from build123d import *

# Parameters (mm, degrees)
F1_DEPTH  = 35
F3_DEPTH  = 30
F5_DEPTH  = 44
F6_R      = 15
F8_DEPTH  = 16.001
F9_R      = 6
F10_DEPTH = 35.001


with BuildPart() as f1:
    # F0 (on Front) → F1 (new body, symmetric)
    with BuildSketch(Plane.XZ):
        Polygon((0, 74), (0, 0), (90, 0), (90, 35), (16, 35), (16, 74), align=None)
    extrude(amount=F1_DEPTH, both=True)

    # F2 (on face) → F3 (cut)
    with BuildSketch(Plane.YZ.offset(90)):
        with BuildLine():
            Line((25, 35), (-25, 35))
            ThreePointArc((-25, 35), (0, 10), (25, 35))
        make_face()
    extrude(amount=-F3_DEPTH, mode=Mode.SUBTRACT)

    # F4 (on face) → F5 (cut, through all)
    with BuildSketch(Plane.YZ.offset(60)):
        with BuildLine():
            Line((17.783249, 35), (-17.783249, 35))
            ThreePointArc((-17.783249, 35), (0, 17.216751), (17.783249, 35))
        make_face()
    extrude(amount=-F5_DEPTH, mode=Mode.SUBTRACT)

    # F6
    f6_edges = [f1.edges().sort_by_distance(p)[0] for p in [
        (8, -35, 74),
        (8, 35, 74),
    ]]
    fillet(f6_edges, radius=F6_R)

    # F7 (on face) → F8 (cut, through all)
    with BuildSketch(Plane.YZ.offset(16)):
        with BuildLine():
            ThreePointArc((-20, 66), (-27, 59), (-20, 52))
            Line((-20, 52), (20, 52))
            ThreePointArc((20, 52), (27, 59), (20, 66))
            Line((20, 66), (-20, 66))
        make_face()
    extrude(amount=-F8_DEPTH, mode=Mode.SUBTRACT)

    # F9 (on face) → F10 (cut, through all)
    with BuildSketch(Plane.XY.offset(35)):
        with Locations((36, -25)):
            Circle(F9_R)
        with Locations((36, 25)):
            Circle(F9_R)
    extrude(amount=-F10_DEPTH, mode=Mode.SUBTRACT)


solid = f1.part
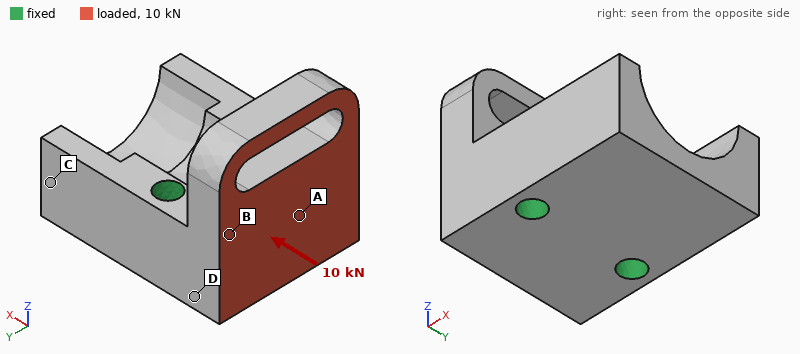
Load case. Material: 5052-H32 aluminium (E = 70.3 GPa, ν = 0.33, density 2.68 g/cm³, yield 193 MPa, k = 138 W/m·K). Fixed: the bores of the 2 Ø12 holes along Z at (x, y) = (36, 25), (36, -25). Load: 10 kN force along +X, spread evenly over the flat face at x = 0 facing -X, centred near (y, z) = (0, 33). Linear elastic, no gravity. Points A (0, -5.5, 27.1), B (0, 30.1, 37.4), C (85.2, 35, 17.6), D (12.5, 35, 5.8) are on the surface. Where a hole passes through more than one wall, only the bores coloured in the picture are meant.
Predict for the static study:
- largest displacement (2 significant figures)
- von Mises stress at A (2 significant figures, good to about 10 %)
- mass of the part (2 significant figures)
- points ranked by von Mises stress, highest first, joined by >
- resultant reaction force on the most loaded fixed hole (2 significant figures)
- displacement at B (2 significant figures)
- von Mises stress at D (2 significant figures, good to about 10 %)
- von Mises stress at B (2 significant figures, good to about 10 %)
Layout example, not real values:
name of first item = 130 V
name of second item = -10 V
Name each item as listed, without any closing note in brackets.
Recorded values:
largest displacement = 0.10 mm
von Mises stress at A = 16 MPa
mass of the part = 510 g
points ranked by von Mises stress, highest first, joined by > = B > A > D > C
resultant reaction force on the most loaded fixed hole = 5.1 kN
displacement at B = 0.019 mm
von Mises stress at D = 7.6 MPa
von Mises stress at B = 31 MPa
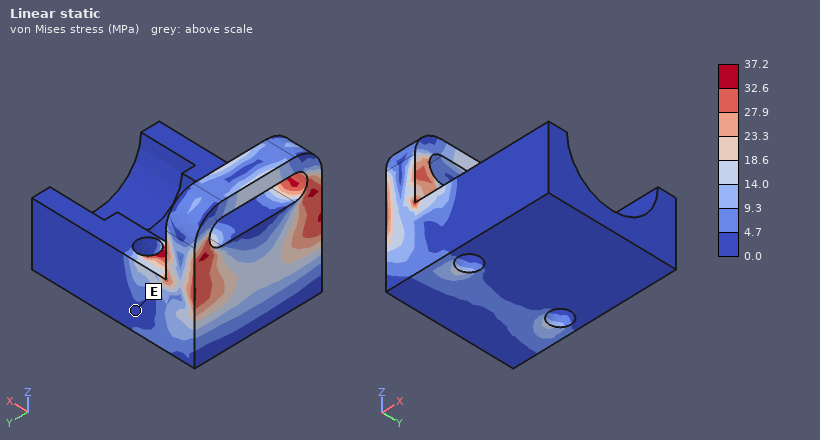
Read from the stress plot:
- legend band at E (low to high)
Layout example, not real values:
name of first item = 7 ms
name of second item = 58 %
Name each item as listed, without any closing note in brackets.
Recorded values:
legend band at E = 0.0 to 4.7 MPa
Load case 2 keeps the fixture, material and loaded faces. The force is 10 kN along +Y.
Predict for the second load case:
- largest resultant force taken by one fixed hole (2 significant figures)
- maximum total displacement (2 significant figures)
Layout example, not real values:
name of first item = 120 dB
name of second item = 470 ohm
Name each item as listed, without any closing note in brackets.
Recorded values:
largest resultant force taken by one fixed hole = 7.9 kN
maximum total displacement = 47 µm
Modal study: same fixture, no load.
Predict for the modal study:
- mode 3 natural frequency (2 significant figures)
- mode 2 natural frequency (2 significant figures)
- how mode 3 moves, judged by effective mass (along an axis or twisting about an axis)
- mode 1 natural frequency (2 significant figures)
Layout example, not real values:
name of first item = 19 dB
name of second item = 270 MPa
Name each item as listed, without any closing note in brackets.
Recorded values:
mode 3 natural frequency = 8500 Hz
mode 2 natural frequency = 6600 Hz
how mode 3 moves, judged by effective mass = twisting about Y
mode 1 natural frequency = 4600 Hz
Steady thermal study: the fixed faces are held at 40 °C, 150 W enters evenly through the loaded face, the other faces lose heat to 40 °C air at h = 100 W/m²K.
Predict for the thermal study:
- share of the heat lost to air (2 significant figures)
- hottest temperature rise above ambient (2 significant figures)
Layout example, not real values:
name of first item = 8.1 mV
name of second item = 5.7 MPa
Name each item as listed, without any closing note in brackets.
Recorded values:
share of the heat lost to air = 13 %
hottest temperature rise above ambient = 31 K
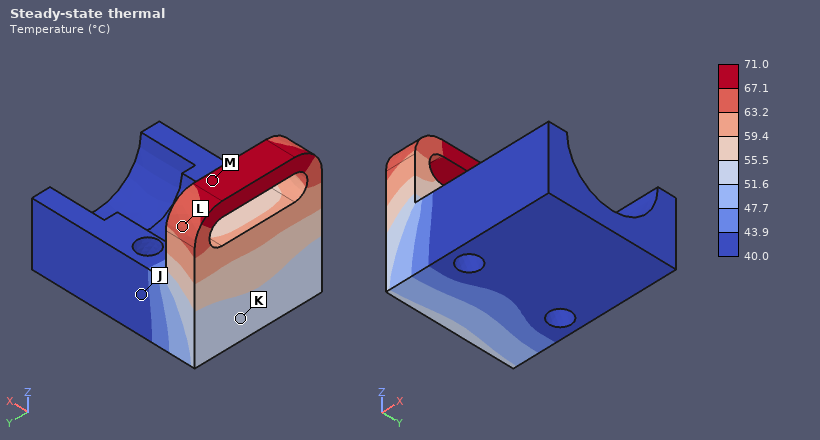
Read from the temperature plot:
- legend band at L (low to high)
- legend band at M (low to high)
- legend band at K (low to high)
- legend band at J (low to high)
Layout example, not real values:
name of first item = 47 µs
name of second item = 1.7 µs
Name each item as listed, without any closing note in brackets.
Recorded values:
legend band at L = 63.2 to 67.1 °C
legend band at M = 67.1 to 71.0 °C
legend band at K = 51.6 to 55.5 °C
legend band at J = 40.0 to 43.9 °C
